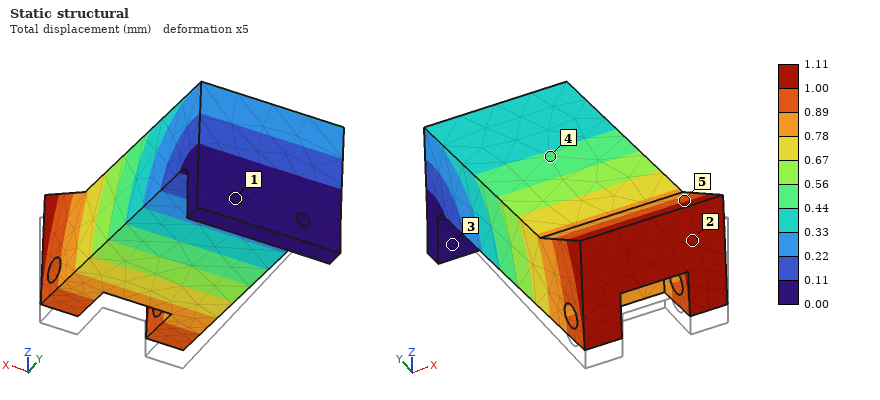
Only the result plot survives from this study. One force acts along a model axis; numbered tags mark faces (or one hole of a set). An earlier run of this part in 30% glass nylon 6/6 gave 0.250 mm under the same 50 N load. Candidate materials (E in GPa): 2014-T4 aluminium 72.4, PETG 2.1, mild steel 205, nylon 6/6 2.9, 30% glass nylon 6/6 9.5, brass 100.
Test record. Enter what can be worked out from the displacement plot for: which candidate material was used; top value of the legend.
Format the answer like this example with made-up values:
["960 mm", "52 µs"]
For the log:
["PETG", "1.11 mm"]
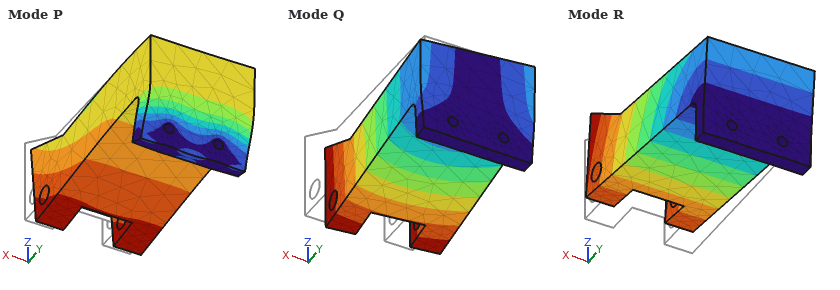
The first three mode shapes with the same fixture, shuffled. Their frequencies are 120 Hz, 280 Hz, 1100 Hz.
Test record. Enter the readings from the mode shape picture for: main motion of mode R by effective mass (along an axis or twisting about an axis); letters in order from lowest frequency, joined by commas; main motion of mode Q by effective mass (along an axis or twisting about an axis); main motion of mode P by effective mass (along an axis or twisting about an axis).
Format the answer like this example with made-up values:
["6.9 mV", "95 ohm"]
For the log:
["along Z", "R, Q, P", "along X", "along Y"]
